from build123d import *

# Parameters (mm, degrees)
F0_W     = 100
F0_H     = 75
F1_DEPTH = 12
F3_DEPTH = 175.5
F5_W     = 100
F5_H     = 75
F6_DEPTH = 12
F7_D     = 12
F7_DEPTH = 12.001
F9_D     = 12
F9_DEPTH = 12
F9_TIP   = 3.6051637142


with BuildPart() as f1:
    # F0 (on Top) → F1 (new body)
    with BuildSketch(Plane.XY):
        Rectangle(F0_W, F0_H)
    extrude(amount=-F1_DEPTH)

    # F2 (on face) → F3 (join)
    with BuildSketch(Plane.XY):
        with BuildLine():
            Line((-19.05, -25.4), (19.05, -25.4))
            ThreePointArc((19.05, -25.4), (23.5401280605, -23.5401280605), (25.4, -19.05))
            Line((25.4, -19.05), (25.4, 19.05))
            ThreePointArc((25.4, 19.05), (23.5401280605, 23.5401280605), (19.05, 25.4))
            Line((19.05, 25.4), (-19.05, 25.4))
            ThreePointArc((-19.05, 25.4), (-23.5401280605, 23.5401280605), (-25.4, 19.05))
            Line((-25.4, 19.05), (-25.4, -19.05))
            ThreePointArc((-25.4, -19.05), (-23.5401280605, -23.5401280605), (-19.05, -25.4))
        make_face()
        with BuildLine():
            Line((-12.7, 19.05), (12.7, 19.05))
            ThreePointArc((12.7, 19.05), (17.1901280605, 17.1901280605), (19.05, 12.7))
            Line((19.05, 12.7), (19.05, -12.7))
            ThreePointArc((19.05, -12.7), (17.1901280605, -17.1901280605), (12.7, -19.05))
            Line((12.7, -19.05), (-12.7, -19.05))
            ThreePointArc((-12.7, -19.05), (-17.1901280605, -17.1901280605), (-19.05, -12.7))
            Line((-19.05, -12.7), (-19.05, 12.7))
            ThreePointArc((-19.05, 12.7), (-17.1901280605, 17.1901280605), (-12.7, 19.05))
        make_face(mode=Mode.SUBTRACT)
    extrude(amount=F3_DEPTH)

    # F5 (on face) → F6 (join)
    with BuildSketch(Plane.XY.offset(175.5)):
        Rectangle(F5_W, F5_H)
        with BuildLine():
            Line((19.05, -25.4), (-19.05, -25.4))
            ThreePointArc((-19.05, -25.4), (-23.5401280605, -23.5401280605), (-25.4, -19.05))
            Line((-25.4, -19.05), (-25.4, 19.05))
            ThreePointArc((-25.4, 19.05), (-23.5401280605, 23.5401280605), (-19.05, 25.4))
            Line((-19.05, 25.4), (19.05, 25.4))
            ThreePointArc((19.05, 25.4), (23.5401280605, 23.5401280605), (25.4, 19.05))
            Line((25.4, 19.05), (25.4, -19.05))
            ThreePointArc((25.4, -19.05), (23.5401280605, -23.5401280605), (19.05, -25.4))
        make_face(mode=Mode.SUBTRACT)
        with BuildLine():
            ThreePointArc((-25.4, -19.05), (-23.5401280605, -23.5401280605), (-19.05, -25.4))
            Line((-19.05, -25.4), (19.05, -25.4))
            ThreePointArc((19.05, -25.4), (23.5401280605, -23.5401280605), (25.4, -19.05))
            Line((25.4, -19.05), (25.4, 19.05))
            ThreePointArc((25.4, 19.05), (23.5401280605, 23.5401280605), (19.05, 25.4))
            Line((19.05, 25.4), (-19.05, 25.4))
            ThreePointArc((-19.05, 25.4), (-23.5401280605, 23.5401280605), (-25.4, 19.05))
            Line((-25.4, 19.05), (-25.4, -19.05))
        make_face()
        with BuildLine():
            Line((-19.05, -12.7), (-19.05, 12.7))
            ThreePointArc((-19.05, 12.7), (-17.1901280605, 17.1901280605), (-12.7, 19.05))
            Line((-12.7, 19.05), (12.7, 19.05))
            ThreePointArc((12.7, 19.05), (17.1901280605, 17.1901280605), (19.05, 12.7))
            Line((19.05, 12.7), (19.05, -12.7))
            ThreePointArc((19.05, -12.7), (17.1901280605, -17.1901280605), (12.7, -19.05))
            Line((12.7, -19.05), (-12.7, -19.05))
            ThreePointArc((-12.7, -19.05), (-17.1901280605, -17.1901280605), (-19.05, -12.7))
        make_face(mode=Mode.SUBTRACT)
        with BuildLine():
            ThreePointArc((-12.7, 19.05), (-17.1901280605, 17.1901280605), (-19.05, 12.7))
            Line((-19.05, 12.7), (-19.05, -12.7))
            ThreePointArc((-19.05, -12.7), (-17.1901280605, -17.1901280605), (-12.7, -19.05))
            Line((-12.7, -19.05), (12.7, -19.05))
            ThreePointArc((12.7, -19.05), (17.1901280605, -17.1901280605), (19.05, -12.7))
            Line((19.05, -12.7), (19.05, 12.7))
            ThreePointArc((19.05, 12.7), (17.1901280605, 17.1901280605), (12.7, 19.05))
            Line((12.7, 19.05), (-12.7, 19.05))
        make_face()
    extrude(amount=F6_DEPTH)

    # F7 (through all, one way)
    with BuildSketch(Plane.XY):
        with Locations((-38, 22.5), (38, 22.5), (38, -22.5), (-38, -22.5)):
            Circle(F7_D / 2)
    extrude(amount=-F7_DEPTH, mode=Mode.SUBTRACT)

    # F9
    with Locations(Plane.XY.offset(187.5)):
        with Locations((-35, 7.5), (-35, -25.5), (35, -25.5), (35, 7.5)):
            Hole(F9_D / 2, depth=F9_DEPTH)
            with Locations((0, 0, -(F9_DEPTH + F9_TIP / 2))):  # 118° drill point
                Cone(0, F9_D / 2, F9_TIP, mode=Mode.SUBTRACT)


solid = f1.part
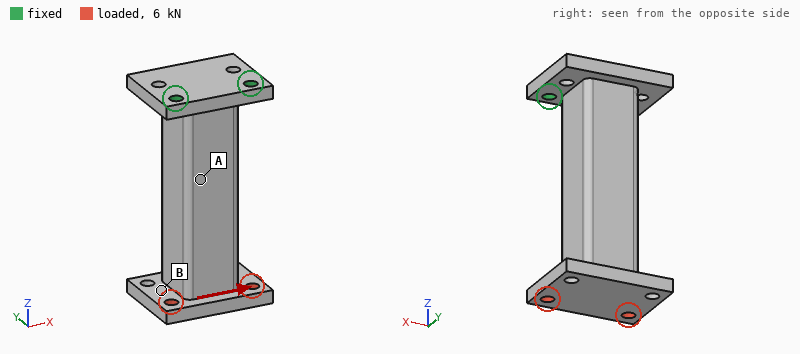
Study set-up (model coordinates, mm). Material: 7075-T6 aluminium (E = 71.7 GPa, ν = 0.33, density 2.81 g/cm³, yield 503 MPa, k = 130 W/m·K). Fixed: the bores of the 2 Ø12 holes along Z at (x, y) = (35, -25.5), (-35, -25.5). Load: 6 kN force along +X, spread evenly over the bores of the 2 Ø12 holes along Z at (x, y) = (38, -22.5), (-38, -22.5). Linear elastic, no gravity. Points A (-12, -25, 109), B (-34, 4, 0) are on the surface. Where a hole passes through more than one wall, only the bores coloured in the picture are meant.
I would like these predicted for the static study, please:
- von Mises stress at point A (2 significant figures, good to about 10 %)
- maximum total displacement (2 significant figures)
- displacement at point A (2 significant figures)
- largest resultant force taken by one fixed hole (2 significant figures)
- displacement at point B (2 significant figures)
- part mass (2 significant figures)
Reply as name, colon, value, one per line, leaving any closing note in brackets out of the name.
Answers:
von Mises stress at point A: 43 MPa
maximum total displacement: 1.1 mm
displacement at point A: 0.29 mm
largest resultant force taken by one fixed hole: 19 kN
displacement at point B: 0.98 mm
part mass: 1.0 kg
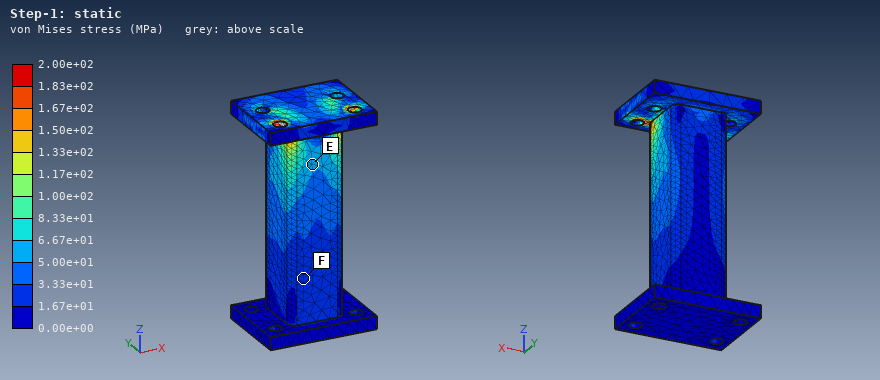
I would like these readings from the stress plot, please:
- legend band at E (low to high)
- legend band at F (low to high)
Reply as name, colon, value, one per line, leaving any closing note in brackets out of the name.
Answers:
legend band at E: 5.00e+01 to 6.67e+01 MPa
legend band at F: 1.67e+01 to 3.33e+01 MPa
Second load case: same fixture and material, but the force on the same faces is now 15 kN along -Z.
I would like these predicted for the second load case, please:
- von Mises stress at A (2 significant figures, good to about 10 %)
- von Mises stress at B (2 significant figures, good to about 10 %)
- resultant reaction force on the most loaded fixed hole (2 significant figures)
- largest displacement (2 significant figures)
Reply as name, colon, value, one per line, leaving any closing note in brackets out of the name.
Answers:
von Mises stress at A: 37 MPa
von Mises stress at B: 47 MPa
resultant reaction force on the most loaded fixed hole: 7.7 kN
largest displacement: 0.44 mm
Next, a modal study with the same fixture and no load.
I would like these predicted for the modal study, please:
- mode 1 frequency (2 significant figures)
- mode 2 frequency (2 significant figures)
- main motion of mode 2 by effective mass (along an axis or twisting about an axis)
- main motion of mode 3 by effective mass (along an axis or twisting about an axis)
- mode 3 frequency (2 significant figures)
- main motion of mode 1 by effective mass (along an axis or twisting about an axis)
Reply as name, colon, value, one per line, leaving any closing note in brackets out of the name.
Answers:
mode 1 frequency: 310 Hz
mode 2 frequency: 620 Hz
main motion of mode 2 by effective mass: along X
main motion of mode 3 by effective mass: twisting about Z
mode 3 frequency: 2300 Hz
main motion of mode 1 by effective mass: along Y
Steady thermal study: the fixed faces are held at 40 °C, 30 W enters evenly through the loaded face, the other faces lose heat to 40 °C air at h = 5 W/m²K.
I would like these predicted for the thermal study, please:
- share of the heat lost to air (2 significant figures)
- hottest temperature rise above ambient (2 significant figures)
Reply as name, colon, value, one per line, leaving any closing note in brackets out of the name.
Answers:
share of the heat lost to air: 28 %
hottest temperature rise above ambient: 40 K
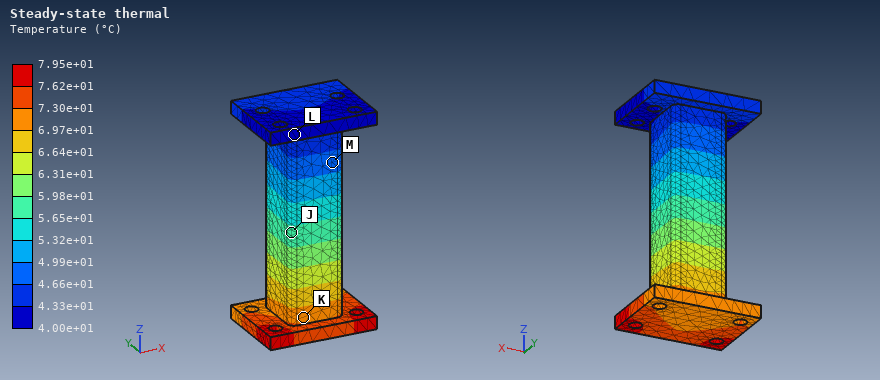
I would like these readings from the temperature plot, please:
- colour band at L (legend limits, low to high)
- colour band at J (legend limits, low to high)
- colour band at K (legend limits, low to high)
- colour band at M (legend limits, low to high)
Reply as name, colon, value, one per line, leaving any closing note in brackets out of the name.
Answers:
colour band at L: 4.00e+01 to 4.33e+01 °C
colour band at J: 5.65e+01 to 5.98e+01 °C
colour band at K: 6.97e+01 to 7.30e+01 °C
colour band at M: 4.66e+01 to 4.99e+01 °C
